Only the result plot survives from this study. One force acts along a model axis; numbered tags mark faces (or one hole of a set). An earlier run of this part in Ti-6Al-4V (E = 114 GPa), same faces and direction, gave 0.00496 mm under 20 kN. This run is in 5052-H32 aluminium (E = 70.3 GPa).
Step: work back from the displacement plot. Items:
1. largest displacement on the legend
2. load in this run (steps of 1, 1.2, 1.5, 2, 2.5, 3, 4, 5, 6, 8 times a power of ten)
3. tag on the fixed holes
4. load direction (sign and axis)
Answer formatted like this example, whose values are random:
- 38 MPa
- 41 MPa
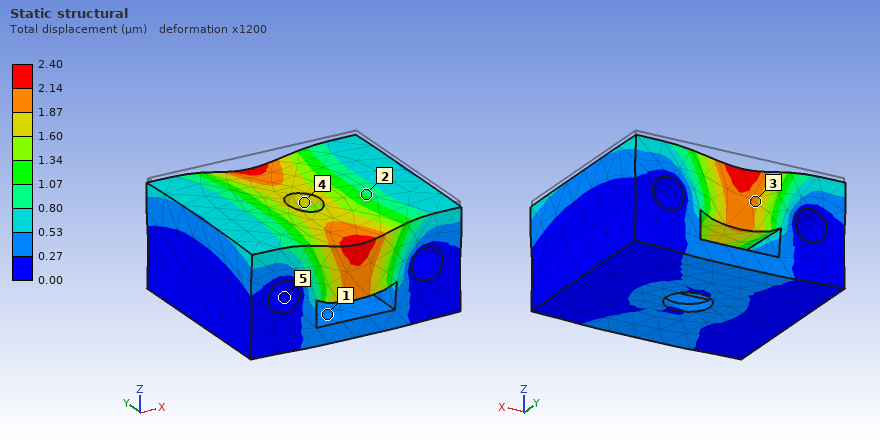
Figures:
- 2.40 µm
- 6 kN
- 5
- -Z
